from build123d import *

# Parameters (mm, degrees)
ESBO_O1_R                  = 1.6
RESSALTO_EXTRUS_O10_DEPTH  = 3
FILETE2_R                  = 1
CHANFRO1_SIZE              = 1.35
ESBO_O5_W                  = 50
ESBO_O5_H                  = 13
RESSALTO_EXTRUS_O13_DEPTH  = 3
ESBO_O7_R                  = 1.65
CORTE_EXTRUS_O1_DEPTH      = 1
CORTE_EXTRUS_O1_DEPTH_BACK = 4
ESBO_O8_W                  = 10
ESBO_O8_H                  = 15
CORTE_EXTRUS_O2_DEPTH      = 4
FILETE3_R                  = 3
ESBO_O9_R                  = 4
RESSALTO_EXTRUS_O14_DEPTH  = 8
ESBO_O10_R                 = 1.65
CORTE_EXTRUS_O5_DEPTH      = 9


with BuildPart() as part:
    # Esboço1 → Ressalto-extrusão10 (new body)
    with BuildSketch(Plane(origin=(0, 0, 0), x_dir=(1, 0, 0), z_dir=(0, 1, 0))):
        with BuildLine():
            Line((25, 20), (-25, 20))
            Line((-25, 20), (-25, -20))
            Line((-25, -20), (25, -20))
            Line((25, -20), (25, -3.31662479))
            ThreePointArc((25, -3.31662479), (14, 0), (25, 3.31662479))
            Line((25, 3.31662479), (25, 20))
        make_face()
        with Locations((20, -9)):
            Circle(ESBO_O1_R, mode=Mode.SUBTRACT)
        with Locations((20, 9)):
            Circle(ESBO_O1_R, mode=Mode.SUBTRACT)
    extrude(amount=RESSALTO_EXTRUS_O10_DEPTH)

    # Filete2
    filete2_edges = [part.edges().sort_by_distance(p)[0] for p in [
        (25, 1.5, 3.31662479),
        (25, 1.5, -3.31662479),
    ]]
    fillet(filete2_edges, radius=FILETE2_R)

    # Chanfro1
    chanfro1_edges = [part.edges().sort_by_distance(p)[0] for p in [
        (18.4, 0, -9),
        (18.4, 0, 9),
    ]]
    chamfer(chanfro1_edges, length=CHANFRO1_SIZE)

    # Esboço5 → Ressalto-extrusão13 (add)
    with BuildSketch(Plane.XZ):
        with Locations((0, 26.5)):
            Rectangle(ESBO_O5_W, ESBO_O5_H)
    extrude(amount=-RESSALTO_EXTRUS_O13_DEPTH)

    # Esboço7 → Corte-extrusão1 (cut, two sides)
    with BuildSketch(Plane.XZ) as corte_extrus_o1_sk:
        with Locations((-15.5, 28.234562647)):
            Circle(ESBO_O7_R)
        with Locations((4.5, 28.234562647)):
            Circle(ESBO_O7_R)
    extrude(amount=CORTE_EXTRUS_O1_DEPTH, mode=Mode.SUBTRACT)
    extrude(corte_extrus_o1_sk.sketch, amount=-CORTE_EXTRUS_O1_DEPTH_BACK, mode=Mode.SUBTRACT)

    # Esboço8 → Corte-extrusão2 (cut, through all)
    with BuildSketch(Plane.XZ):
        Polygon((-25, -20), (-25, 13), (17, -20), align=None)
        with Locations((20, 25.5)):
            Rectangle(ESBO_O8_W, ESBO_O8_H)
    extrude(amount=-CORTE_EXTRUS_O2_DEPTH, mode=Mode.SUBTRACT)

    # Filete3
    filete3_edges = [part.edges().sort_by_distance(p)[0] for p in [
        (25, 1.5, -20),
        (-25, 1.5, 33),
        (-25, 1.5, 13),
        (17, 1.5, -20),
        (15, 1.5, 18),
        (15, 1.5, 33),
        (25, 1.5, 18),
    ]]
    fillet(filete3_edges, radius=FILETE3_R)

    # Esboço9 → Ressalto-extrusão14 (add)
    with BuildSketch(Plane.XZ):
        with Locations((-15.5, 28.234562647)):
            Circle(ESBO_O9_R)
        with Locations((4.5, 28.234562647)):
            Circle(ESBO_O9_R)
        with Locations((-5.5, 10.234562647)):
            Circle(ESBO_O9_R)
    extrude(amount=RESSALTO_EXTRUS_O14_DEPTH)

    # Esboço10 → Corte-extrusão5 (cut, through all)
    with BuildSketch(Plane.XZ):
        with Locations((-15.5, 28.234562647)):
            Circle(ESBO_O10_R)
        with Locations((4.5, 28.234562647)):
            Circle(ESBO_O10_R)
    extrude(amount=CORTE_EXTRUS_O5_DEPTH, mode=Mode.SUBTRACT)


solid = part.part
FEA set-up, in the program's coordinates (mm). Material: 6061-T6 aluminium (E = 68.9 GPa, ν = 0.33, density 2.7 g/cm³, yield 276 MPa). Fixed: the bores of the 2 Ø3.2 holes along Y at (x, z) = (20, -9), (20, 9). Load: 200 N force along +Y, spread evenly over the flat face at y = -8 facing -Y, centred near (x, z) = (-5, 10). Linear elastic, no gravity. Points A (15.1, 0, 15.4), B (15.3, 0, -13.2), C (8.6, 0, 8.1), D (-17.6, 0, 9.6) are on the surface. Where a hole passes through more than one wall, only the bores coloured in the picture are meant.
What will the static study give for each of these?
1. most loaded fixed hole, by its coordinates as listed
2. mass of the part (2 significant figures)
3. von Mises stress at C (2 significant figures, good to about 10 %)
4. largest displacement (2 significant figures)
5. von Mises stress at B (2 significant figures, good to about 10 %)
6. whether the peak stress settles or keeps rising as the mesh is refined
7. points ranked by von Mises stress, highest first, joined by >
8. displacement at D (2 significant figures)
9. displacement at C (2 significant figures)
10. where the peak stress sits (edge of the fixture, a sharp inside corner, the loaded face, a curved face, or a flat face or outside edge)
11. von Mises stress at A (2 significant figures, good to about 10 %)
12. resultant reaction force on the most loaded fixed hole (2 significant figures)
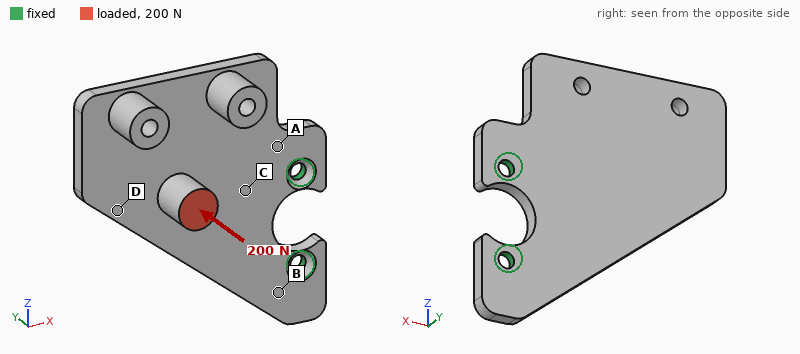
(20, 9)
16 g
48 MPa
0.82 mm
80 MPa
keeps rising
A > B > C > D
0.62 mm
0.13 mm
edge of the fixture
110 MPa
180 N
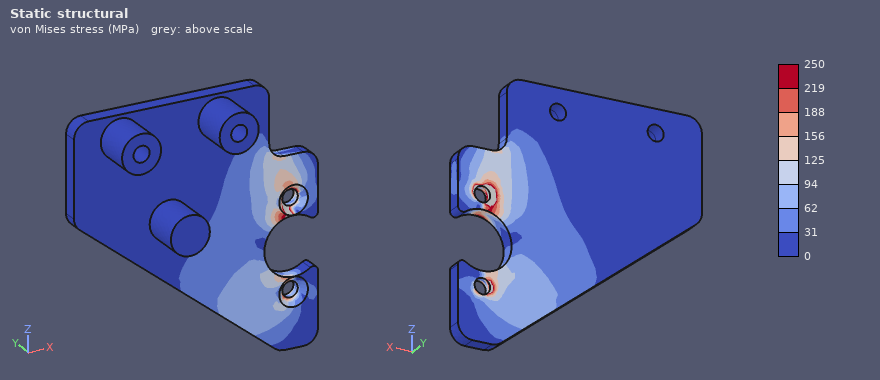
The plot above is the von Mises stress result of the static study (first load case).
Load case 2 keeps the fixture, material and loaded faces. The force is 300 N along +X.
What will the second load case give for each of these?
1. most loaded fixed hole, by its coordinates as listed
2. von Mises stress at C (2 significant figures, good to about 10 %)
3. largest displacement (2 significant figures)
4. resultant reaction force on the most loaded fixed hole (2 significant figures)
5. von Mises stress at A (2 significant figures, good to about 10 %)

(20, 9)
54 MPa
0.63 mm
290 N
87 MPa
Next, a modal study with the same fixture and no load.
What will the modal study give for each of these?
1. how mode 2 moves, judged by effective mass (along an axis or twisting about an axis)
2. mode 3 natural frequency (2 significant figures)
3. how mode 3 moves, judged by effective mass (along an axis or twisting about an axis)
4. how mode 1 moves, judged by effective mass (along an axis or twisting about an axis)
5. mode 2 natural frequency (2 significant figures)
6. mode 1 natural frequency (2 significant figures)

twisting about X
4900 Hz
along Y
along Y
2700 Hz
840 Hz
